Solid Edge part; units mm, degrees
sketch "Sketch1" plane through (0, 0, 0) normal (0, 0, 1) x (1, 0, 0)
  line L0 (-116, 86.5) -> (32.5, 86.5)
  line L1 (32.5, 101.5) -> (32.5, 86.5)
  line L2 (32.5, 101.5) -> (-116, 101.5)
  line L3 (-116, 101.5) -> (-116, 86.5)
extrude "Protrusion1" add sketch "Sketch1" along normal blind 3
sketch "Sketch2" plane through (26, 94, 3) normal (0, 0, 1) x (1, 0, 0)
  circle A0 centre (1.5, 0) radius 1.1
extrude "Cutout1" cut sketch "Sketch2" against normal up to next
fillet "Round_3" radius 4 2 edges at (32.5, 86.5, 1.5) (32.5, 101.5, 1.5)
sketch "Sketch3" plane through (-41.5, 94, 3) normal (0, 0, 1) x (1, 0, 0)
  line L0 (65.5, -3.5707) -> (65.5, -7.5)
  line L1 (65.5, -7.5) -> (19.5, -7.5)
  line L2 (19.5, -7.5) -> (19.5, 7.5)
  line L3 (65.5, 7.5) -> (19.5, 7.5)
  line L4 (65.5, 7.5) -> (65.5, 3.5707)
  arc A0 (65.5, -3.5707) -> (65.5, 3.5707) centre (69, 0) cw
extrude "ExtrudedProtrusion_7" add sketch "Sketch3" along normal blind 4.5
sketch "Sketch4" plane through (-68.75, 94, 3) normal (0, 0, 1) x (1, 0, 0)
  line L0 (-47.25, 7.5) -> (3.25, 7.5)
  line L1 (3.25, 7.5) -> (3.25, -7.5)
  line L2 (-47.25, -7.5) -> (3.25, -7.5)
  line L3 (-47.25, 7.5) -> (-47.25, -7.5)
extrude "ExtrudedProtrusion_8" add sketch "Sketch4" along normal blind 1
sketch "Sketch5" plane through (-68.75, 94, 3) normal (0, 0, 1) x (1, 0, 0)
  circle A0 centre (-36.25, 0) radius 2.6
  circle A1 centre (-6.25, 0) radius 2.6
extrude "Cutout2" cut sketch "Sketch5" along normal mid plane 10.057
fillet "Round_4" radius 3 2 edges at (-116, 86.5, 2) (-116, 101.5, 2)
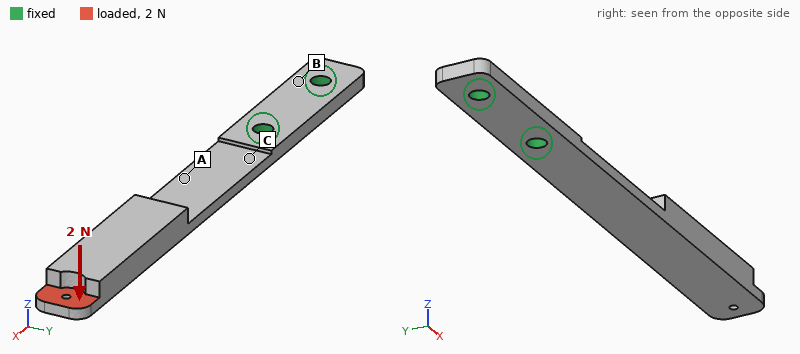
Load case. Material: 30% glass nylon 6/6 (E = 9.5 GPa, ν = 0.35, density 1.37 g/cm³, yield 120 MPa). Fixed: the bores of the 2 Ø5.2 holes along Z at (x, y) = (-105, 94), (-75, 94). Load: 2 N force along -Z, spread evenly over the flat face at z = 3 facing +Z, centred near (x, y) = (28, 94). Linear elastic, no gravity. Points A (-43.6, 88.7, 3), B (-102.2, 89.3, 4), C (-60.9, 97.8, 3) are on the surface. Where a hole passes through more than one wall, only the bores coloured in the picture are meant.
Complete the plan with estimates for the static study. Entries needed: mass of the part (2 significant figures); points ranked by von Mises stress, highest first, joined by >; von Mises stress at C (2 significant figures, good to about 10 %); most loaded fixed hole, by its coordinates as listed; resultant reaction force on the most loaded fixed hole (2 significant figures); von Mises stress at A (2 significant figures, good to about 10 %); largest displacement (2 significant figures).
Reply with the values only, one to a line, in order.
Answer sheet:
14 g
C > A > B
7.7 MPa
(-75, 94)
2.1 N
6.3 MPa
1.8 mm
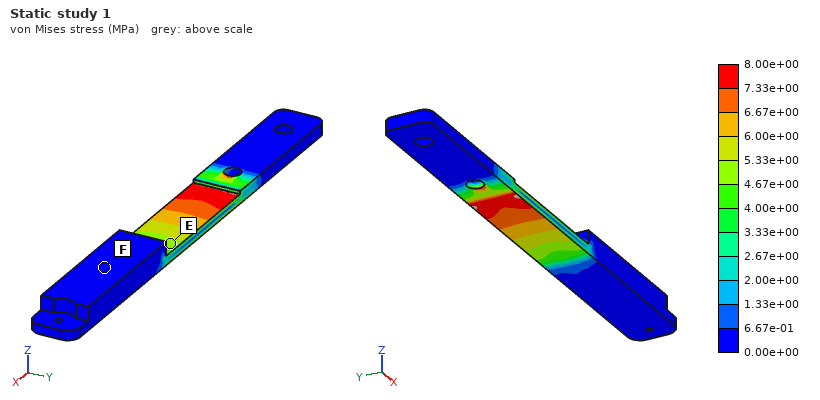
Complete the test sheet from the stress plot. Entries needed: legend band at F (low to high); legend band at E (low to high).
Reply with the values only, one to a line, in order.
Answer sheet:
0.00e+00 to 6.67e-01 MPa
4.67e+00 to 5.33e+00 MPa
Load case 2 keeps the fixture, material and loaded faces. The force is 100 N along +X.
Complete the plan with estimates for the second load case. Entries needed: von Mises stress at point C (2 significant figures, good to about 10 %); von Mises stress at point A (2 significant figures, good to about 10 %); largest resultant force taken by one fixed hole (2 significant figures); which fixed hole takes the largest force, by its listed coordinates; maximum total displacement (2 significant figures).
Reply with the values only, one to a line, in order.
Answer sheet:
8.7 MPa
8.9 MPa
95 N
(-75, 94)
1.7 mm
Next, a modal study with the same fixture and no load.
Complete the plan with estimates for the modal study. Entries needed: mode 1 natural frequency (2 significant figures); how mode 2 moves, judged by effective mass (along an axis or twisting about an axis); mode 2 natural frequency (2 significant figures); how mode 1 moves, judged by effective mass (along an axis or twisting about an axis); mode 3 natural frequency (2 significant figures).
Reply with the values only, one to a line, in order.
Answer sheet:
90 Hz
along Y
380 Hz
along Z
860 Hz
